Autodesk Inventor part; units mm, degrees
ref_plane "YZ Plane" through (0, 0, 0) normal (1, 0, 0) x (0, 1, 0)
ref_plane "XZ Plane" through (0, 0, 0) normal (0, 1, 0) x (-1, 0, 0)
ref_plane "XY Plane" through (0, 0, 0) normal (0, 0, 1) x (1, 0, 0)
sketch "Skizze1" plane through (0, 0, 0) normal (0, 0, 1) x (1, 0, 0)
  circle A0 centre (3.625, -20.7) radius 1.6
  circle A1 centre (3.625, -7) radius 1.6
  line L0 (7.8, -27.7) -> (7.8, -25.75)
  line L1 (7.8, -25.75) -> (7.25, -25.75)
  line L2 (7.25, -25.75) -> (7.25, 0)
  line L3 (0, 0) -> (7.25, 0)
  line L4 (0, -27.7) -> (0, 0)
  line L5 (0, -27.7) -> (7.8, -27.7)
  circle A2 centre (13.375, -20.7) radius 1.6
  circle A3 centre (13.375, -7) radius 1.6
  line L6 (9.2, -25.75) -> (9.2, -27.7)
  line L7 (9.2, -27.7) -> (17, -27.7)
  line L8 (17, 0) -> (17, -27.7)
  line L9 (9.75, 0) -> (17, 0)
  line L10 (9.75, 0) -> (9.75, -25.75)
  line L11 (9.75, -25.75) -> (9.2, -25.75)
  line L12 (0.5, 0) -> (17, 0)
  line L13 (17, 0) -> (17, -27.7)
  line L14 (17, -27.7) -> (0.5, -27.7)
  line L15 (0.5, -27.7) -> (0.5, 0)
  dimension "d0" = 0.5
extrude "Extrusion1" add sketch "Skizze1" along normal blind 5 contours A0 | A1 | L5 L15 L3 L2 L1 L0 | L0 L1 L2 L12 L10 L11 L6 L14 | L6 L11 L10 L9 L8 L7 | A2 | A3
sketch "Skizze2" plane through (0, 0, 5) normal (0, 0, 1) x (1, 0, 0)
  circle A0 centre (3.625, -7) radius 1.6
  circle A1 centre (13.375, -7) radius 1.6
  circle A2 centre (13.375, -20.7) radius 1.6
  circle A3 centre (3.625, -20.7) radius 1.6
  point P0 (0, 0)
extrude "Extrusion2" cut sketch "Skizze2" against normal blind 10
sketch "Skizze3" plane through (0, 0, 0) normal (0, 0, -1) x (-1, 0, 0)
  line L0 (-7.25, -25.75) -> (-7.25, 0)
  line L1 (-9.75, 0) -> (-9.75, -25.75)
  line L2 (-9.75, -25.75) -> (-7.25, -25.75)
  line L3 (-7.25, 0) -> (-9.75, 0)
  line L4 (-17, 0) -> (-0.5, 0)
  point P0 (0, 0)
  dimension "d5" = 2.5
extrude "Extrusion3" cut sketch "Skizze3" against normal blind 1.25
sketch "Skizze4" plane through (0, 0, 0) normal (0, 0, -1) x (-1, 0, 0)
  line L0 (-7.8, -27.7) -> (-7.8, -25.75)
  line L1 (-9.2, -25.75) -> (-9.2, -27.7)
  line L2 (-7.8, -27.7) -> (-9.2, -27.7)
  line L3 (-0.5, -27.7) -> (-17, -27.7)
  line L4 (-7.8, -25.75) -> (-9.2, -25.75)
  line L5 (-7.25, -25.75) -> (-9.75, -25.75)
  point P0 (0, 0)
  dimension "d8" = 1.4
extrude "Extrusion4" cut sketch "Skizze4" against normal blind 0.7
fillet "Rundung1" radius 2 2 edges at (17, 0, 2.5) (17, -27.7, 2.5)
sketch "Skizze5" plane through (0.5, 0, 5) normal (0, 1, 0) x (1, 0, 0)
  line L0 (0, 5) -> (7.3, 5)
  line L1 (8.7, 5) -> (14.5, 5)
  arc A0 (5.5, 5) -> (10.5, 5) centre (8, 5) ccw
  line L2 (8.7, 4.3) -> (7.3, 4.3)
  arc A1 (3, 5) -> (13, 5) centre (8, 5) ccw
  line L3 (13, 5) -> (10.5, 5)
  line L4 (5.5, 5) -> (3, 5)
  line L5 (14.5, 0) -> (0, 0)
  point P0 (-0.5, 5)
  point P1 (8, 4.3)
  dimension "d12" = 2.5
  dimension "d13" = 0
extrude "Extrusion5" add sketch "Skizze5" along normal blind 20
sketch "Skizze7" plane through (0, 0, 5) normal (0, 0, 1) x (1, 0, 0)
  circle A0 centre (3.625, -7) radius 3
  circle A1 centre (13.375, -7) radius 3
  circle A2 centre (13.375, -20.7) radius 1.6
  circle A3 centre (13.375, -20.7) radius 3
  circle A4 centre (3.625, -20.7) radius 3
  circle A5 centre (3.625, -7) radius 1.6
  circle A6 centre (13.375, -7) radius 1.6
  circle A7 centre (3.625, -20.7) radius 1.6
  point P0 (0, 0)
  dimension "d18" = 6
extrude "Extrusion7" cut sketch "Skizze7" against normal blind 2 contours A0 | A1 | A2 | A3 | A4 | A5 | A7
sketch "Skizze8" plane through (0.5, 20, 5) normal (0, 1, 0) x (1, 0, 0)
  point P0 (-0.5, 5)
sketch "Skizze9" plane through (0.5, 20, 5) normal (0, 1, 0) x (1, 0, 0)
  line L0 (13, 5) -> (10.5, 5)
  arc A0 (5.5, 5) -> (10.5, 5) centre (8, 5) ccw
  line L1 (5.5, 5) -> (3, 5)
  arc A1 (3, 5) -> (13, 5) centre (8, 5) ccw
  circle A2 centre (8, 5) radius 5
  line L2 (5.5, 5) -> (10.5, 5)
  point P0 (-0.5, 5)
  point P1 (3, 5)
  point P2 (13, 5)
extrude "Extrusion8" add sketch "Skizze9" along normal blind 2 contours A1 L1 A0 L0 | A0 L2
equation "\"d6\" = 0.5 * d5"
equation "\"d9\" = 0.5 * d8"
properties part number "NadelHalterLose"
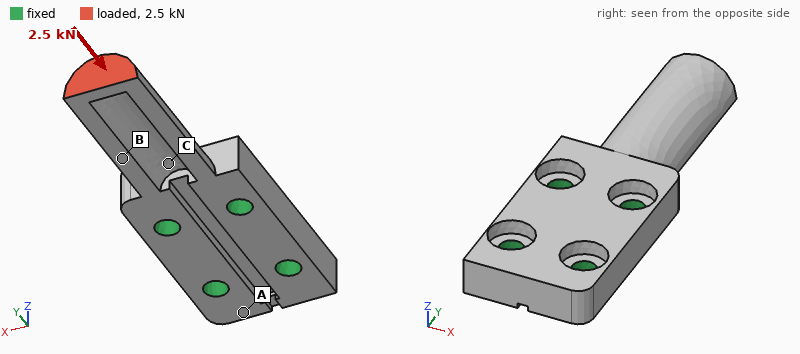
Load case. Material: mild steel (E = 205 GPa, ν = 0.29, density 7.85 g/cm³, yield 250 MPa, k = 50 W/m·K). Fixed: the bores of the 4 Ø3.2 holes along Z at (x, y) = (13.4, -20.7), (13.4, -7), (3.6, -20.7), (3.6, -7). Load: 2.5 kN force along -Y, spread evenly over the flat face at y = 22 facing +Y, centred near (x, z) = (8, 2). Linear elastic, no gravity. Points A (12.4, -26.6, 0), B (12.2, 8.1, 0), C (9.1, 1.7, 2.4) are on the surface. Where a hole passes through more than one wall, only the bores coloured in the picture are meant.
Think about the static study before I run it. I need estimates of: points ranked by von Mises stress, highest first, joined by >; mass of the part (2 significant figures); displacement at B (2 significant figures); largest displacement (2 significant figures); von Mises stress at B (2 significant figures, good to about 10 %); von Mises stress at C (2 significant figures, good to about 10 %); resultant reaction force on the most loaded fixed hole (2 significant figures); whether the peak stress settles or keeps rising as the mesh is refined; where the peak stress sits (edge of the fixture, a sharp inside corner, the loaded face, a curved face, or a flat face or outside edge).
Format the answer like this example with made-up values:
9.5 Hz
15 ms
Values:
B > C > A
20 g
7.0 µm
27 µm
130 MPa
78 MPa
1.2 kN
keeps rising
a sharp inside corner
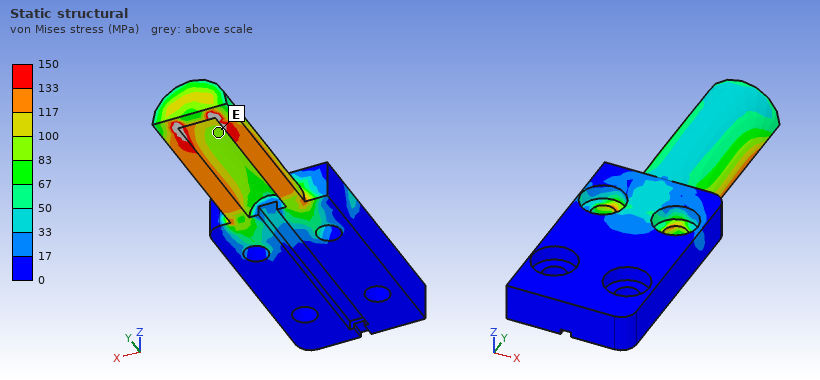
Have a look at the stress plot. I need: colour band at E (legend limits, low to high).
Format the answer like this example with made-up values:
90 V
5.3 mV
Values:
83 to 100 MPa
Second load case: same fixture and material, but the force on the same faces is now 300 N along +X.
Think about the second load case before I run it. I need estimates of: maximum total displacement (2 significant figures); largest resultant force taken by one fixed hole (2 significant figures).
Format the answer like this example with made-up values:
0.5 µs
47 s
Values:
50 µm
760 N
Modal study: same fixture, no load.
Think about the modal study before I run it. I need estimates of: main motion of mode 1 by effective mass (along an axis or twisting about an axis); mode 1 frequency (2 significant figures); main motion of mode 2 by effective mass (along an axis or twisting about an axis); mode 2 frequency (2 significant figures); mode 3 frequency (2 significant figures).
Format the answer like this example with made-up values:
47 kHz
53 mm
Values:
along Z
4800 Hz
along X
10 kHz
17 kHz
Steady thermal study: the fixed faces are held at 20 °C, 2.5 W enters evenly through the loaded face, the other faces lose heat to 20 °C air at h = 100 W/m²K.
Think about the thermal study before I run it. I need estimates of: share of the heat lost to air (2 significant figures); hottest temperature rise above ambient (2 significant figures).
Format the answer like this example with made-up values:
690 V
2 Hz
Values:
44 %
31 K
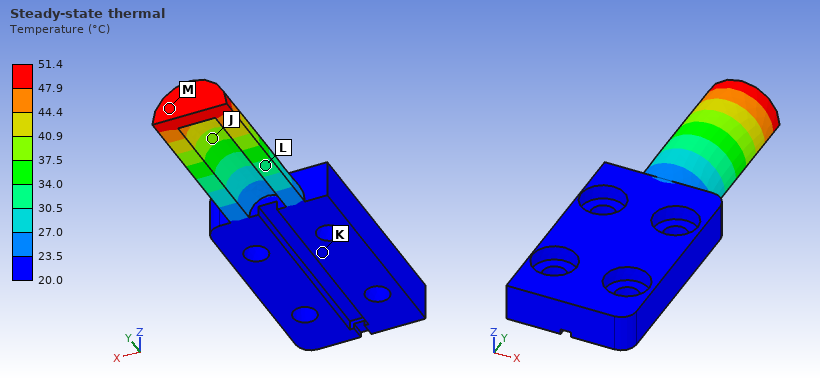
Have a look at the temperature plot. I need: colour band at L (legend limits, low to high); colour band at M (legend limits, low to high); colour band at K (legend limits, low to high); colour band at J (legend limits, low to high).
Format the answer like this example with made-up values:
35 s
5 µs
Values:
30.5 to 34.0 °C
47.9 to 51.4 °C
20.0 to 23.5 °C
37.5 to 40.9 °C
